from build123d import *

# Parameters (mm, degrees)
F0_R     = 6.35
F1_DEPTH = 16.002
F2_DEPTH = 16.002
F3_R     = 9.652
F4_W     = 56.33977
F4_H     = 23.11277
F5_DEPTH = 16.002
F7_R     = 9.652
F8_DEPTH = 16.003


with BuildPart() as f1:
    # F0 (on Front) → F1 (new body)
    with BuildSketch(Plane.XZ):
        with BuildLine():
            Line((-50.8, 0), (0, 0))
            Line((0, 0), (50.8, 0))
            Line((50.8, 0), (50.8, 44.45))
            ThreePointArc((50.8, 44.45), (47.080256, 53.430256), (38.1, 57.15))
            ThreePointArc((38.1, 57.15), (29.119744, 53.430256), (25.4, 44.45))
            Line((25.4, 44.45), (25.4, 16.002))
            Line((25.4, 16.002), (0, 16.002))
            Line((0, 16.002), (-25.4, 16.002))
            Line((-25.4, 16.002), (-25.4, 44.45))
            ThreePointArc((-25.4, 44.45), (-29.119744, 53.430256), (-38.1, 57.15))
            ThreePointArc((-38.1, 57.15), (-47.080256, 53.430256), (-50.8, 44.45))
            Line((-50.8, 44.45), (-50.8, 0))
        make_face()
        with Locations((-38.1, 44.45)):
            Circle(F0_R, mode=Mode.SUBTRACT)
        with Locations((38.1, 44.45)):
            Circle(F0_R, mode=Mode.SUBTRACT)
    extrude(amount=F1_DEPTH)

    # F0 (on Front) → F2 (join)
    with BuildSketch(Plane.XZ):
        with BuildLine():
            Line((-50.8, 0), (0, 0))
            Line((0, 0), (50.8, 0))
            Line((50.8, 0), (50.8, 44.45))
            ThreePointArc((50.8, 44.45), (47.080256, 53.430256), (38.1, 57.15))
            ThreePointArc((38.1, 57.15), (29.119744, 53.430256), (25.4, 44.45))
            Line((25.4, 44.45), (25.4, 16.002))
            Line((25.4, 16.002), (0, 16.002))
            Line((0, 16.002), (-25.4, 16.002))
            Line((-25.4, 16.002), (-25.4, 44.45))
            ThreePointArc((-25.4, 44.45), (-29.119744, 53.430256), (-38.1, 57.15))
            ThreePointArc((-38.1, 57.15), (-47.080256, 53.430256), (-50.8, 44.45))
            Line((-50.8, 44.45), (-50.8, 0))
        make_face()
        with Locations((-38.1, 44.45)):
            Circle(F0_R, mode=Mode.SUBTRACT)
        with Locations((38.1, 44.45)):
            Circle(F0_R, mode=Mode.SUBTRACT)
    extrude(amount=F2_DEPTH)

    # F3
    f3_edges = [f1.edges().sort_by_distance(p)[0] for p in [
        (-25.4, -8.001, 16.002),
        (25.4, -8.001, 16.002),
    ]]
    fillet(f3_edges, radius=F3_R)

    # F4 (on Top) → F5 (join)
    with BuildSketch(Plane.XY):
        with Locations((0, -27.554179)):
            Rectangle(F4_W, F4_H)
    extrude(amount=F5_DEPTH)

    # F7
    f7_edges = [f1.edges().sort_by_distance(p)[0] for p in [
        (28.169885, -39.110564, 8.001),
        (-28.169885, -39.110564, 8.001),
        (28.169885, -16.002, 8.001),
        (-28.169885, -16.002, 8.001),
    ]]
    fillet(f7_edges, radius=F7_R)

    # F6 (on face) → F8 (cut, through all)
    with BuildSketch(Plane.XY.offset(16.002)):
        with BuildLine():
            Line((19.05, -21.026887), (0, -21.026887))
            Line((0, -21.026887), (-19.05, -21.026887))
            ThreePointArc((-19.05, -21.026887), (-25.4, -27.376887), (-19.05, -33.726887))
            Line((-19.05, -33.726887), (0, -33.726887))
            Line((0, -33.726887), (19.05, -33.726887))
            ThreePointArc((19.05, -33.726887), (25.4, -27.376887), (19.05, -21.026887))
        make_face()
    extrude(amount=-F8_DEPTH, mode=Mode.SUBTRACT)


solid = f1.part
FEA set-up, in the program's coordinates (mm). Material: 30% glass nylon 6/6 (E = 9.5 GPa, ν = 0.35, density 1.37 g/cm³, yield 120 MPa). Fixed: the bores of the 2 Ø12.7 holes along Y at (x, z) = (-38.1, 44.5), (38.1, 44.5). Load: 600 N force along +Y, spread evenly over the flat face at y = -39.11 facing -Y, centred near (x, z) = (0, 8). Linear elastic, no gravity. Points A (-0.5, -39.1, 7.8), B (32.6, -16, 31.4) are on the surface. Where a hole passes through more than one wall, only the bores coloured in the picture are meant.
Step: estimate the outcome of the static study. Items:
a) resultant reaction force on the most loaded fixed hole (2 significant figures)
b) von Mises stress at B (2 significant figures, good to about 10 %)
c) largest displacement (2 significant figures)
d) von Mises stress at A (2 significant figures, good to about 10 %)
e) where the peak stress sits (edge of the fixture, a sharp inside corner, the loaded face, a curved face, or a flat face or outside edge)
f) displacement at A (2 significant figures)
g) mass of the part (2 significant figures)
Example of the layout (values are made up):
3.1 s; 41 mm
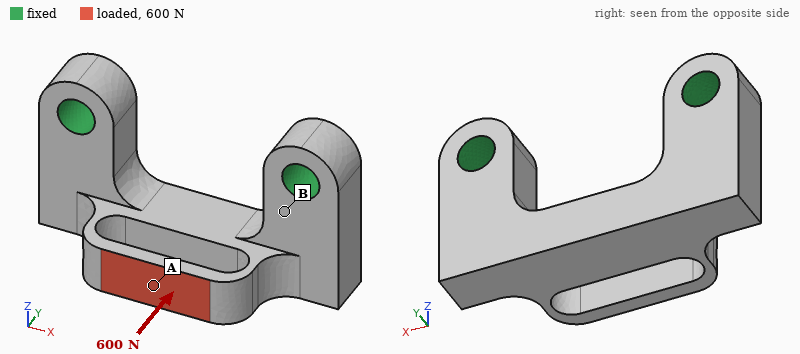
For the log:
300 N; 6.6 MPa; 0.36 mm; 33 MPa; a curved face; 0.33 mm; 89 g
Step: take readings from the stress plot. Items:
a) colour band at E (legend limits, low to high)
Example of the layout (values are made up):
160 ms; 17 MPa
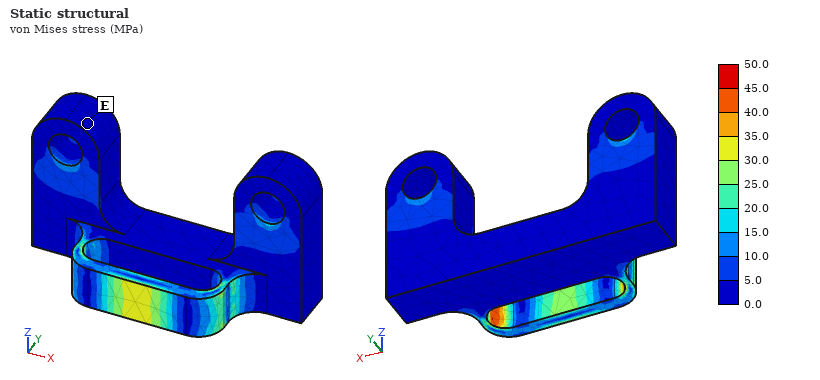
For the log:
0.0 to 5.0 MPa
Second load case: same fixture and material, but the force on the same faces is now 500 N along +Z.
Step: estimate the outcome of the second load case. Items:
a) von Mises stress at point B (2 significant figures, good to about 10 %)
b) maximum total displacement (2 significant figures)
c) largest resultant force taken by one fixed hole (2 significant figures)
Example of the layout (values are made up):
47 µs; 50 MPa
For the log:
8.4 MPa; 0.34 mm; 270 N
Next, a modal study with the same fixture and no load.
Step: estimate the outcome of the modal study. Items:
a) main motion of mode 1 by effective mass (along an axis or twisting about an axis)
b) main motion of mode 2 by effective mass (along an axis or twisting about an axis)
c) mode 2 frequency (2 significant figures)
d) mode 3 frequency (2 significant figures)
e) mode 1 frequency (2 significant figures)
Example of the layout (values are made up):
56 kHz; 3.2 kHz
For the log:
along Y; along X; 3100 Hz; 3700 Hz; 2000 Hz
